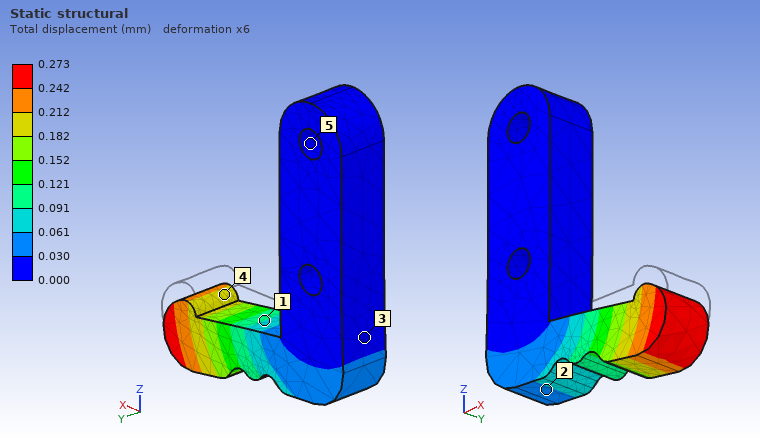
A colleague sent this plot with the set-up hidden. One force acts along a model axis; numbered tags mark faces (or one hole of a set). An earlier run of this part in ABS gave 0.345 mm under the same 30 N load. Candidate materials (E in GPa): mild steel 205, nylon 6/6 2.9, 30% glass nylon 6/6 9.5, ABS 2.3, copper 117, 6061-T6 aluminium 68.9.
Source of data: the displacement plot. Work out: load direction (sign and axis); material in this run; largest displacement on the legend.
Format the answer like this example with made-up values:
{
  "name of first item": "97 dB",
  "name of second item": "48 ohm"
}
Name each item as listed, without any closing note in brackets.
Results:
{
  "load direction": "-Z",
  "material in this run": "nylon 6/6",
  "largest displacement on the legend": "0.273 mm"
}
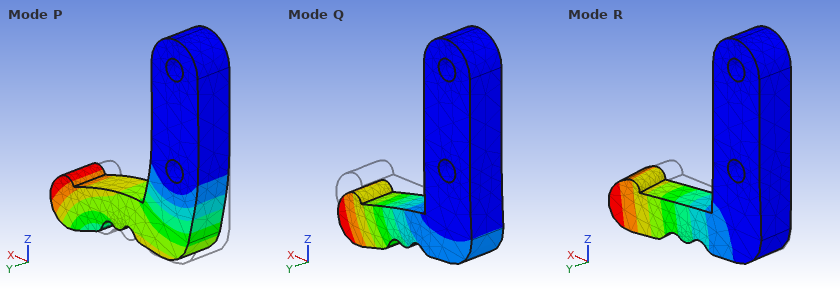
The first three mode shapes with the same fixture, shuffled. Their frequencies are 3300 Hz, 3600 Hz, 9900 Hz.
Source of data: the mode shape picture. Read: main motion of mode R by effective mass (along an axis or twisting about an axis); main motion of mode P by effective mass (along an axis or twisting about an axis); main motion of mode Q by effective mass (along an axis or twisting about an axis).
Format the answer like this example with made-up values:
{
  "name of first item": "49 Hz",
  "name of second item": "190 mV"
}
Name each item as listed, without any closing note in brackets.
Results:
{
  "main motion of mode R by effective mass": "along Y",
  "main motion of mode P by effective mass": "along X",
  "main motion of mode Q by effective mass": "along Z"
}
